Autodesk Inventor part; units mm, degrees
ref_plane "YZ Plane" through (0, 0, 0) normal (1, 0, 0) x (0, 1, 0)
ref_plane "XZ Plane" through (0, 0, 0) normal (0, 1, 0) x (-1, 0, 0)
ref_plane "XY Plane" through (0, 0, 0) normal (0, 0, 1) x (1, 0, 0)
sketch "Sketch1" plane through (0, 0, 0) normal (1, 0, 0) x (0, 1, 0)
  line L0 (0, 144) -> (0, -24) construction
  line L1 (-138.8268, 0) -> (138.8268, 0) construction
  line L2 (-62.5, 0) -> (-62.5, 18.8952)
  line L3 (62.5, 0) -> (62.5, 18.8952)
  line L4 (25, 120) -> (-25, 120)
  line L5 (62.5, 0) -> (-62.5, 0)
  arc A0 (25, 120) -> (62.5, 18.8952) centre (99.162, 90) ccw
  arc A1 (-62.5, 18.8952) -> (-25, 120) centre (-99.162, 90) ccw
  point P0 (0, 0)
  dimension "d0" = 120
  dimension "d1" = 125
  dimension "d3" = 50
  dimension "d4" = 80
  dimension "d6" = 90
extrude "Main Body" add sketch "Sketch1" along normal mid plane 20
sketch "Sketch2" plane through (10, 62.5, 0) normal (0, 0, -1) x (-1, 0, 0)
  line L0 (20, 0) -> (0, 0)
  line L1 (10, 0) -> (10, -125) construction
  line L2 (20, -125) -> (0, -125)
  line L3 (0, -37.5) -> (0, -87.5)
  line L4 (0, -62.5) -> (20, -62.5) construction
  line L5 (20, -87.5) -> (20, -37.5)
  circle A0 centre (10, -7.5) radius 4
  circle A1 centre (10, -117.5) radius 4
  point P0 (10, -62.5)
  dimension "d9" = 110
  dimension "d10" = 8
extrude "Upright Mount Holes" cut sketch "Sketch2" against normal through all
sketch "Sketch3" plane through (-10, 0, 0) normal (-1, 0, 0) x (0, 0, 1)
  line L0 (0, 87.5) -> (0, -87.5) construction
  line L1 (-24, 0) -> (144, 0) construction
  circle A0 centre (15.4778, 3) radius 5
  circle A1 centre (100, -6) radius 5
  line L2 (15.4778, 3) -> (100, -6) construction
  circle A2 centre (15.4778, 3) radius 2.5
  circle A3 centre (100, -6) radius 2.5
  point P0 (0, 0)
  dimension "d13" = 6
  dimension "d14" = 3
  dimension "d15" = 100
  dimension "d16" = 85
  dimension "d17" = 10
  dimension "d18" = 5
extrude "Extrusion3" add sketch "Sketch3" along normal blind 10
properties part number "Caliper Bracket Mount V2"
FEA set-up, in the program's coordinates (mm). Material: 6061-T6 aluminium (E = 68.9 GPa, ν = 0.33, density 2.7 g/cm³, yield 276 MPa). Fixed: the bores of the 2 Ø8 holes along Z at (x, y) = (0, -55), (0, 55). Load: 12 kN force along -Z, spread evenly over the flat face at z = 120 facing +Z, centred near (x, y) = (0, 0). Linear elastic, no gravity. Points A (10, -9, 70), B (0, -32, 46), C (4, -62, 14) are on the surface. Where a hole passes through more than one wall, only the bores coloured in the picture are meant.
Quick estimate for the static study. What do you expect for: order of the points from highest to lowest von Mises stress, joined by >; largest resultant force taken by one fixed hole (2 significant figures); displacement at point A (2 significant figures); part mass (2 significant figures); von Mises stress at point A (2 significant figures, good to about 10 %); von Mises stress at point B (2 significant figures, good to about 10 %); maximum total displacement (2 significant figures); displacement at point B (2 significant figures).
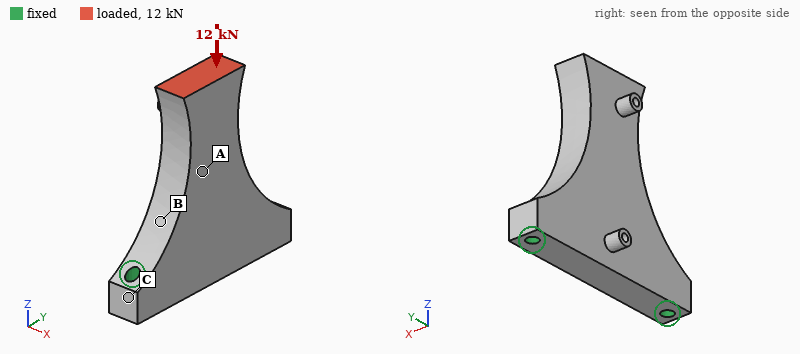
B > A > C
6.9 kN
21 µm
440 g
13 MPa
21 MPa
36 µm
14 µm
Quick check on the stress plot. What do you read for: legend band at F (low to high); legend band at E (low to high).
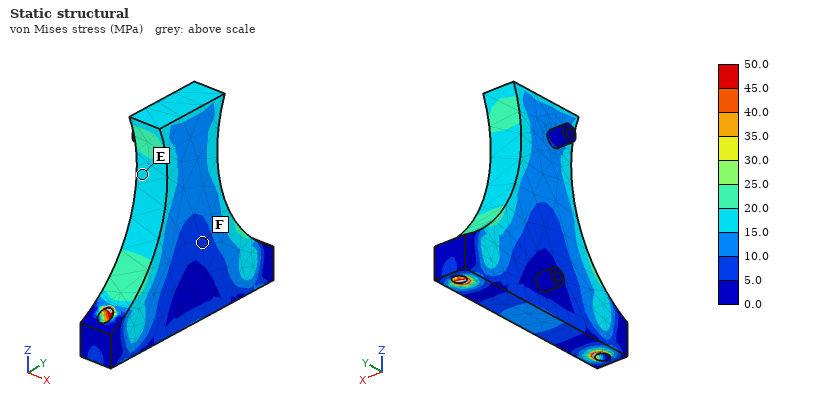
5.0 to 10.0 MPa
15.0 to 20.0 MPa
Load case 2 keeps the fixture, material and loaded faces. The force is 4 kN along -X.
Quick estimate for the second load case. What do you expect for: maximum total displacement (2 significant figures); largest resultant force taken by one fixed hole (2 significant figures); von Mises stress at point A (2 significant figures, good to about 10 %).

0.97 mm
2.0 kN
71 MPa
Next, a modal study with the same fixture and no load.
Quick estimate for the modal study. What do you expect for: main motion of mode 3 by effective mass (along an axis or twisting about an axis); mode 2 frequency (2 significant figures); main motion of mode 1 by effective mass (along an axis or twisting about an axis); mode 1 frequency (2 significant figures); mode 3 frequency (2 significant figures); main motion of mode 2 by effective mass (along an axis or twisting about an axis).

along X
4500 Hz
along X
1200 Hz
5200 Hz
along Y
